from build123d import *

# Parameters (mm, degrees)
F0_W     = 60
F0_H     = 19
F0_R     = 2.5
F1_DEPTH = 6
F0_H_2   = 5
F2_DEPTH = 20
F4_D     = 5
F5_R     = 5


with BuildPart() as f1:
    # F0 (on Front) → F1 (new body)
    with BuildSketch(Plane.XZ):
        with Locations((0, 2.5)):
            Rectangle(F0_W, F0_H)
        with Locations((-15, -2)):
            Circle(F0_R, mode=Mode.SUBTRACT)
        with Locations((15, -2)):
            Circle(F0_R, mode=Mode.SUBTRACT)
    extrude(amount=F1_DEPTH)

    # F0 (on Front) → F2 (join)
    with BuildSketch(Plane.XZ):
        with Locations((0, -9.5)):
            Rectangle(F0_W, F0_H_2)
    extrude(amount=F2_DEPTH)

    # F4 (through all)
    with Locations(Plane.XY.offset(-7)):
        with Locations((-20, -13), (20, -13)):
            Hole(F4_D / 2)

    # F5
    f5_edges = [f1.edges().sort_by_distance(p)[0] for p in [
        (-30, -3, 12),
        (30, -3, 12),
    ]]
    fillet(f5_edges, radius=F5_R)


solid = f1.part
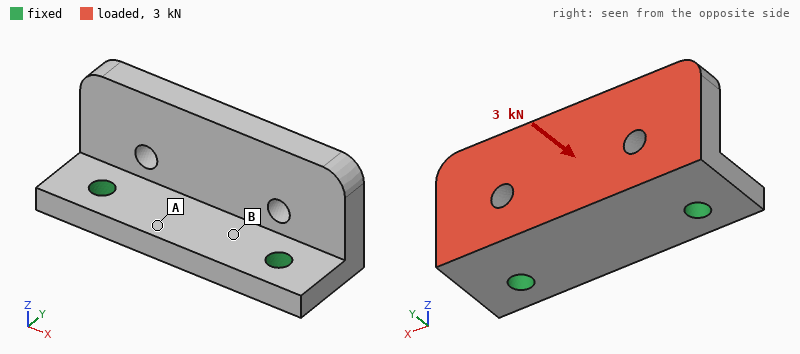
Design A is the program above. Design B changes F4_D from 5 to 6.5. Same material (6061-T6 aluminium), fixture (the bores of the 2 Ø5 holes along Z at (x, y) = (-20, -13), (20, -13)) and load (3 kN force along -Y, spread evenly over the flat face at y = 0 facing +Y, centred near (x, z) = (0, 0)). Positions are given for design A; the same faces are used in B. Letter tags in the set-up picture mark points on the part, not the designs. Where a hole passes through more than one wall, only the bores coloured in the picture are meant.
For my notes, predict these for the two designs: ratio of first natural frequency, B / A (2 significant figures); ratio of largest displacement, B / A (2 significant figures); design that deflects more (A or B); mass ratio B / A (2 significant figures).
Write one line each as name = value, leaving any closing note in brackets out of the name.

ratio of first natural frequency, B / A = 1.1
ratio of largest displacement, B / A = 0.88
design that deflects more = A
mass ratio B / A = 0.99
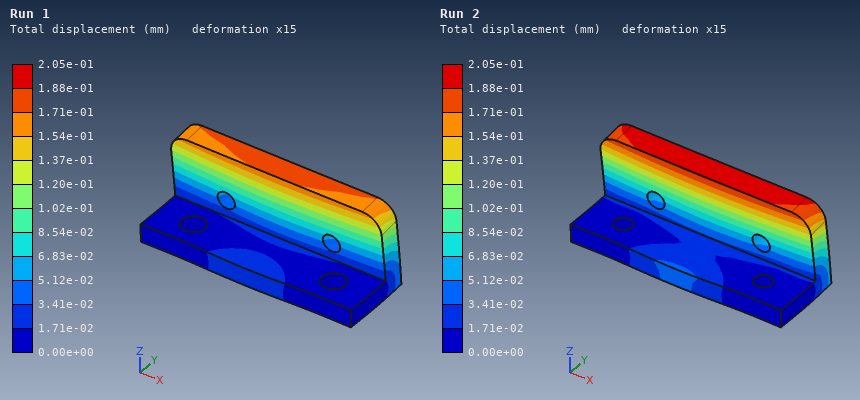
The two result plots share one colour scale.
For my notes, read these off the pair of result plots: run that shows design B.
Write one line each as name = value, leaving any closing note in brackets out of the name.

run that shows design B = Run 1
